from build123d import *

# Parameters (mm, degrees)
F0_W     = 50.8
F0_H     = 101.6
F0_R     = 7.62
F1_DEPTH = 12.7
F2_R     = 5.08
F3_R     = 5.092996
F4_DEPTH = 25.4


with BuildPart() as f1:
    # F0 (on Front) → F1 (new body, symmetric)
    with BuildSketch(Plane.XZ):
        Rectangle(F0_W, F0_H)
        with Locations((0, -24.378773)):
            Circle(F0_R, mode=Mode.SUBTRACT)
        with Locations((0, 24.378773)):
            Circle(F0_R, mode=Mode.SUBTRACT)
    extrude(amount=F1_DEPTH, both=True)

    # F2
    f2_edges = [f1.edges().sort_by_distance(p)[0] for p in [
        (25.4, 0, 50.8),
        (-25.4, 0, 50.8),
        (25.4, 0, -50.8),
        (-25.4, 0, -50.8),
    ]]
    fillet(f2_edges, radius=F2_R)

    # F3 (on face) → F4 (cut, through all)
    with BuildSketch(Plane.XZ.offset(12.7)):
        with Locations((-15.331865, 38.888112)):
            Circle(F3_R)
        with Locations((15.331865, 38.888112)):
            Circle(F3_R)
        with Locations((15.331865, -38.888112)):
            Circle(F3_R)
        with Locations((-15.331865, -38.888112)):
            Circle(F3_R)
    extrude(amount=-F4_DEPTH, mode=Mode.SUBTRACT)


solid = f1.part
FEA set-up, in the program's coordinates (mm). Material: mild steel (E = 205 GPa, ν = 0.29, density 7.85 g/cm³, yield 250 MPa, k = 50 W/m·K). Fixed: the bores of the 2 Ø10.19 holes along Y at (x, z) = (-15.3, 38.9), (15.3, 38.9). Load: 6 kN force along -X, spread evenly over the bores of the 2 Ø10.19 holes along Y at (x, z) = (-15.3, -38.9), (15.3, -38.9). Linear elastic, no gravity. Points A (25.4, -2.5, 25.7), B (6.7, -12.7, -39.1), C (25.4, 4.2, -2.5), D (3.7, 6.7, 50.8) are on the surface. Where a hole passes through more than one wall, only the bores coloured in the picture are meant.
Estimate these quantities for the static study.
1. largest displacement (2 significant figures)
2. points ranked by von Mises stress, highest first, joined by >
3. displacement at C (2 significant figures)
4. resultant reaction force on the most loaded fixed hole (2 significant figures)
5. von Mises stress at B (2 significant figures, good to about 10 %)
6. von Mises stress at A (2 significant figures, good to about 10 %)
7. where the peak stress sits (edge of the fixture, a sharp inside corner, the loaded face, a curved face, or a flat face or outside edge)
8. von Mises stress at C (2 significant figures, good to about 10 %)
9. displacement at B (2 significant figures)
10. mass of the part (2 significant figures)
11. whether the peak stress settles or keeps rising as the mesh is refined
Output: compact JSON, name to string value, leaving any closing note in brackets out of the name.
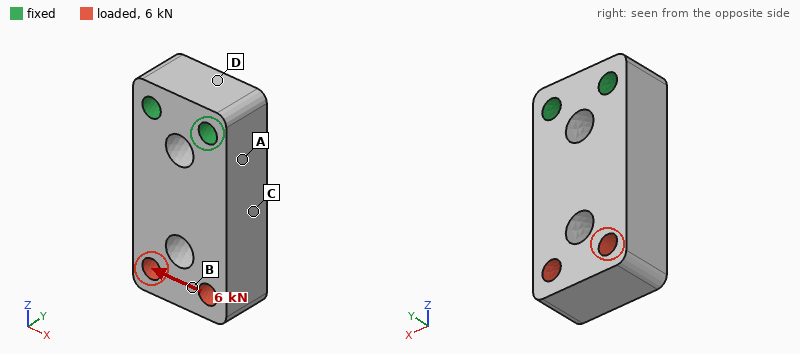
{"largest displacement": "29 µm", "points ranked by von Mises stress, highest first, joined by >": "A > C > B > D", "displacement at C": "12 µm", "resultant reaction force on the most loaded fixed hole": "12 kN", "von Mises stress at B": "12 MPa", "von Mises stress at A": "33 MPa", "where the peak stress sits": "edge of the fixture", "von Mises stress at C": "21 MPa", "displacement at B": "24 µm", "mass of the part": "890 g", "whether the peak stress settles or keeps rising as the mesh is refined": "keeps rising"}
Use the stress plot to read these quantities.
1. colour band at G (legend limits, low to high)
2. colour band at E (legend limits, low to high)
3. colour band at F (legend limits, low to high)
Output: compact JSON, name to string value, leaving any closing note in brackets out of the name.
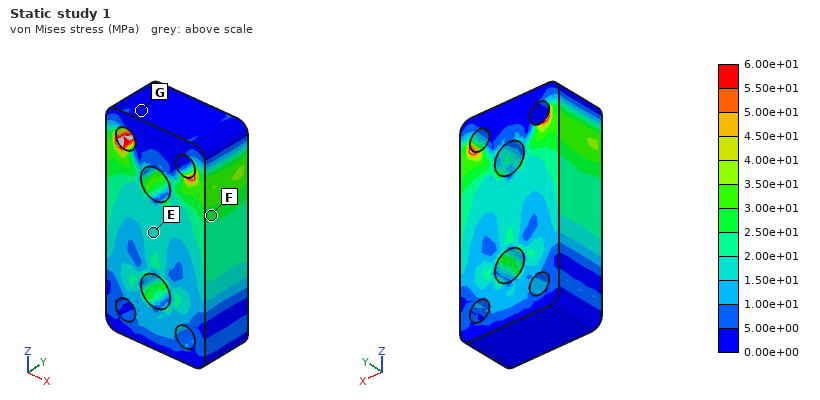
{"colour band at G": "0.00e+00 to 5.00e+00 MPa", "colour band at E": "1.50e+01 to 2.00e+01 MPa", "colour band at F": "2.50e+01 to 3.00e+01 MPa"}
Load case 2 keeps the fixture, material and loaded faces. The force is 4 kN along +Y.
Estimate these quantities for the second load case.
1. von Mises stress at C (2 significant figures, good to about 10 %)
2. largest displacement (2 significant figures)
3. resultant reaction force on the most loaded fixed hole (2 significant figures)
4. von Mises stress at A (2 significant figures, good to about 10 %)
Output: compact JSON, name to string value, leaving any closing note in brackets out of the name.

{"von Mises stress at C": "15 MPa", "largest displacement": "67 µm", "resultant reaction force on the most loaded fixed hole": "2.0 kN", "von Mises stress at A": "9.9 MPa"}
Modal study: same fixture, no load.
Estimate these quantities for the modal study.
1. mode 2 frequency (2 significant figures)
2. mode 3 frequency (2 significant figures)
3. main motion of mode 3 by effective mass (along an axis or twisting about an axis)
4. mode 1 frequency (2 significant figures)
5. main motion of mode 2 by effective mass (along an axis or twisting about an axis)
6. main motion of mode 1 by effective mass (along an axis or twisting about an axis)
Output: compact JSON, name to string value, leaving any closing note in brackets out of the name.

{"mode 2 frequency": "4500 Hz", "mode 3 frequency": "7000 Hz", "main motion of mode 3 by effective mass": "twisting about Z", "mode 1 frequency": "2500 Hz", "main motion of mode 2 by effective mass": "along X", "main motion of mode 1 by effective mass": "along Y"}
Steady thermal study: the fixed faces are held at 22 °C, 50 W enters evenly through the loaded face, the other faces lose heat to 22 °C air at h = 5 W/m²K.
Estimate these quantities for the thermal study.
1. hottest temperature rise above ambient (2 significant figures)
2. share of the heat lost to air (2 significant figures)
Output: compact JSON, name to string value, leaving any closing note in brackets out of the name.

{"hottest temperature rise above ambient": "71 K", "share of the heat lost to air": "6.1 %"}
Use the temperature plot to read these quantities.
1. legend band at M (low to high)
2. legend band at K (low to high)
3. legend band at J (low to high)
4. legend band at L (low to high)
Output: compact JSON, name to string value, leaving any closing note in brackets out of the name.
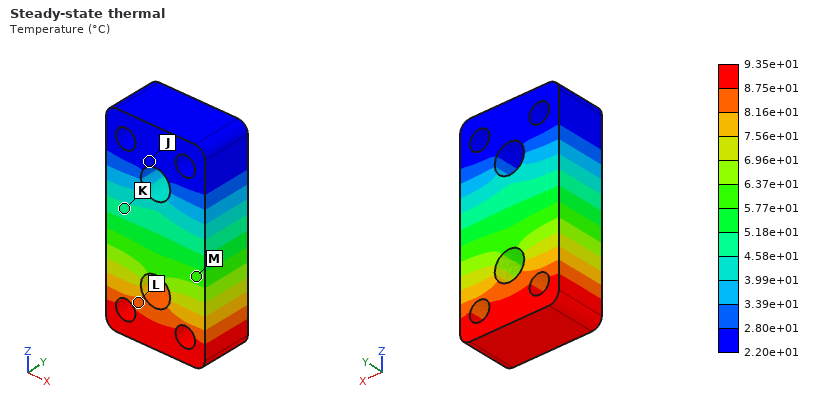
{"legend band at M": "5.77e+01 to 6.37e+01 °C", "legend band at K": "4.58e+01 to 5.18e+01 °C", "legend band at J": "2.20e+01 to 2.80e+01 °C", "legend band at L": "8.16e+01 to 8.75e+01 °C"}
